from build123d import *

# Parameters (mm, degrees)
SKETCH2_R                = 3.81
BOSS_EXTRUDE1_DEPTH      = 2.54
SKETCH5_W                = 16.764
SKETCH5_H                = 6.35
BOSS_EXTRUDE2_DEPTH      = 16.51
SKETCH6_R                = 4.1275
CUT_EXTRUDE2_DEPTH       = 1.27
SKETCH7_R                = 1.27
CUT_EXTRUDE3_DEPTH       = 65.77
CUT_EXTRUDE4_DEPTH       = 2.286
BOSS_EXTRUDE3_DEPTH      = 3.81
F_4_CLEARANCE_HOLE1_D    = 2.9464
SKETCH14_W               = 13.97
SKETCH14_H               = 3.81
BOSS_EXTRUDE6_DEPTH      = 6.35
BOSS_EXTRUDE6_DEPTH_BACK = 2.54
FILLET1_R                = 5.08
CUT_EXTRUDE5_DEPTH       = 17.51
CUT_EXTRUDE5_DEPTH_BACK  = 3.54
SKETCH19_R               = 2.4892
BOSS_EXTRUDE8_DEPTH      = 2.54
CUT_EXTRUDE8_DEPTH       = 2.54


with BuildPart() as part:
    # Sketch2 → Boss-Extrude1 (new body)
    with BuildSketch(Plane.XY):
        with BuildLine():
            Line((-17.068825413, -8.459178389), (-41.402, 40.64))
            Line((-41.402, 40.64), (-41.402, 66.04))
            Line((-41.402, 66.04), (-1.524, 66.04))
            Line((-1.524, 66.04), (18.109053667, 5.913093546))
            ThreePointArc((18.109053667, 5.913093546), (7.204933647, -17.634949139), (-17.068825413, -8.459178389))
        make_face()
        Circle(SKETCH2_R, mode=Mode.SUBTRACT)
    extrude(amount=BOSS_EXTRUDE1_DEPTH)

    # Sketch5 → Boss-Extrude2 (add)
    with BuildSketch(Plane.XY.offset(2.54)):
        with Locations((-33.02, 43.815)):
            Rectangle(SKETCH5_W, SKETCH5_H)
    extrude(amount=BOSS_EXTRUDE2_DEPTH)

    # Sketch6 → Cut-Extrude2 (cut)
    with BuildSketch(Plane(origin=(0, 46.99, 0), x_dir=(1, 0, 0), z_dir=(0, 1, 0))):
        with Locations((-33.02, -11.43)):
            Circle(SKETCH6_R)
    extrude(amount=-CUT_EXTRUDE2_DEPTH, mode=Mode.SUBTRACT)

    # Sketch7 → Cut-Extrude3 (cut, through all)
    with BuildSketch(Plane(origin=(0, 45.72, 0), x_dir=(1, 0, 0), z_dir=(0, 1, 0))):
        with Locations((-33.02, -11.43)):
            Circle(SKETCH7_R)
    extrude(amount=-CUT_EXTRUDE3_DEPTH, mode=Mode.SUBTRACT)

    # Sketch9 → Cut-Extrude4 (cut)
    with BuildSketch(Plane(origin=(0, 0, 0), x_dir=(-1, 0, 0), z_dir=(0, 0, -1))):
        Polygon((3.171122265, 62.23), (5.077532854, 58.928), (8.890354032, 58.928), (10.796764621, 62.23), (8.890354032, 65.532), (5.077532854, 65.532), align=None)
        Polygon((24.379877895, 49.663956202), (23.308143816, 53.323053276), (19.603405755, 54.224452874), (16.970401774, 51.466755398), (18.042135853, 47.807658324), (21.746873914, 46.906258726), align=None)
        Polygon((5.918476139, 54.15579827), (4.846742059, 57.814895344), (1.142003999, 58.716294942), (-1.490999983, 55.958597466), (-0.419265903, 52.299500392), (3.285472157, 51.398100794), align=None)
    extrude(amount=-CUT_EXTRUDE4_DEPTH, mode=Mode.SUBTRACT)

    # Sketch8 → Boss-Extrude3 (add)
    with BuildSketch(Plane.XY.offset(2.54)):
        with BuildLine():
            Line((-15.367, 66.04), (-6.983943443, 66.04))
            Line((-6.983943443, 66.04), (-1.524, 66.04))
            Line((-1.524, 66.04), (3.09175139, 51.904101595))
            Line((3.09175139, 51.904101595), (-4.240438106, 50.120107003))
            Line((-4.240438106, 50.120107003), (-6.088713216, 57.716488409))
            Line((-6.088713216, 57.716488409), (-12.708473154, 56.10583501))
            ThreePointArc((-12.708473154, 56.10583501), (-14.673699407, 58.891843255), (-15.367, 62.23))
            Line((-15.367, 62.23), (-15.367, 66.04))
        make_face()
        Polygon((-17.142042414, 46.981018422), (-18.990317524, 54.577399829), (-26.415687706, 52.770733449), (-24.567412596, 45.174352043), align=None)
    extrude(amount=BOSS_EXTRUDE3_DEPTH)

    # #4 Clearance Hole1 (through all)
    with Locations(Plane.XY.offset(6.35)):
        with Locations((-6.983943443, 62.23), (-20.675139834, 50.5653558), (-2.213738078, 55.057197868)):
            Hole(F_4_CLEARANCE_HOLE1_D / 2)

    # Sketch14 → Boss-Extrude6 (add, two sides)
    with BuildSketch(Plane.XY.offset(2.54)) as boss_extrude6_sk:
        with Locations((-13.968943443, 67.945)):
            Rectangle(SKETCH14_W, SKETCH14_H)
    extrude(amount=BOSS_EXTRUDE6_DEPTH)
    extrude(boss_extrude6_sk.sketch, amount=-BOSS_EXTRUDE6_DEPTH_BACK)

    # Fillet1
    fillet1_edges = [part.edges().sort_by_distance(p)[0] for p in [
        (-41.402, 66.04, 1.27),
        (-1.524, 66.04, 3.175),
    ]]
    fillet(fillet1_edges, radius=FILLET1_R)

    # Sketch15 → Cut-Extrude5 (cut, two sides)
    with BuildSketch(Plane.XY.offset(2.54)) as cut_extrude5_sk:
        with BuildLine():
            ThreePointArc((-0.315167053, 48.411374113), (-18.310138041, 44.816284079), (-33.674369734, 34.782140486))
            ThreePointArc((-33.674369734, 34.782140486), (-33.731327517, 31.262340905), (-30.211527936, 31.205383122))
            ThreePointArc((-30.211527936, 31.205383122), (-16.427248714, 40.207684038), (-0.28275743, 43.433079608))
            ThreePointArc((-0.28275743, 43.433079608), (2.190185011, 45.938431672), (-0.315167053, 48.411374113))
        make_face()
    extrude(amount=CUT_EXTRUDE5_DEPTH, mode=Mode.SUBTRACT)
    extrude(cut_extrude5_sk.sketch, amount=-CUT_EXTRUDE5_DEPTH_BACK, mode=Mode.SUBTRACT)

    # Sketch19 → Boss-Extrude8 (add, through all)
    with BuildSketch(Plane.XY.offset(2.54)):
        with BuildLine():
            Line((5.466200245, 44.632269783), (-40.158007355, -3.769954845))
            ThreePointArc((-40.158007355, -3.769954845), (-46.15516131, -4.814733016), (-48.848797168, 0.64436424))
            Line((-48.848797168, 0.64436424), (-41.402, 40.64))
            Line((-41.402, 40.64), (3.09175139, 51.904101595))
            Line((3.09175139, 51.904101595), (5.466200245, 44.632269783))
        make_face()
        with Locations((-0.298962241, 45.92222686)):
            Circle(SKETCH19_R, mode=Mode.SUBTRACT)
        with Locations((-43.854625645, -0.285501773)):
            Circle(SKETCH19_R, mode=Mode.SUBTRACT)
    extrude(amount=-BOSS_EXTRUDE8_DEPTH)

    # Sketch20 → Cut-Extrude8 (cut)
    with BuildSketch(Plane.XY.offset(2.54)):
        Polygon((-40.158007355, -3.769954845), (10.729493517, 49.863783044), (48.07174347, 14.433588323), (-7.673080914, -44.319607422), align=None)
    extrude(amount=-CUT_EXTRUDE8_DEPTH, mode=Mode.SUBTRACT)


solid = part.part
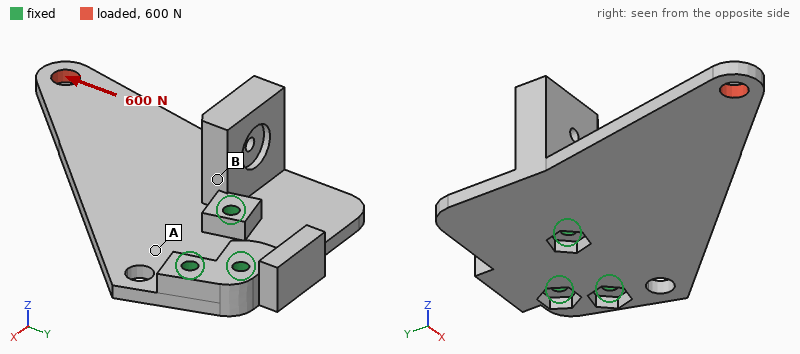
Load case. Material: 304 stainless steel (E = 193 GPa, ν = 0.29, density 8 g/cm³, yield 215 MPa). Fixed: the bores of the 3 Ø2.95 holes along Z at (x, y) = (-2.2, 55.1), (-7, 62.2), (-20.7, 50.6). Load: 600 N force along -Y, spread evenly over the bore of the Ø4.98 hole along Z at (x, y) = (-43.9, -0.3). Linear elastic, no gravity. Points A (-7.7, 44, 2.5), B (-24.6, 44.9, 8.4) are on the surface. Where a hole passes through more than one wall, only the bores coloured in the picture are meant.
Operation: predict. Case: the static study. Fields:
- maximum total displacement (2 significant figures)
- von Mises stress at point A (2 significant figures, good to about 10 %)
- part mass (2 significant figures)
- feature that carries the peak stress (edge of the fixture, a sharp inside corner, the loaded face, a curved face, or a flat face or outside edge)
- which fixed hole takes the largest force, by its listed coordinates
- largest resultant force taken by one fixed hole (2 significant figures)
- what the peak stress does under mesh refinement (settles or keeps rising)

45 µm
22 MPa
67 g
edge of the fixture
(-20.7, 50.6)
970 N
keeps rising
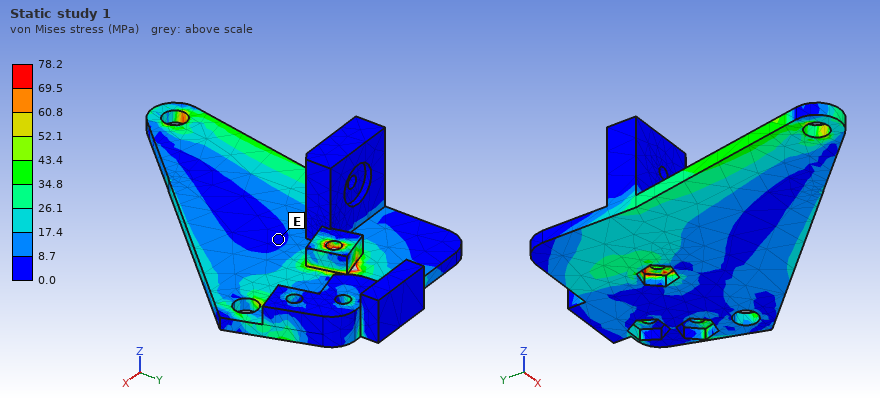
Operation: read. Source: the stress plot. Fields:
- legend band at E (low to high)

0.0 to 8.7 MPa
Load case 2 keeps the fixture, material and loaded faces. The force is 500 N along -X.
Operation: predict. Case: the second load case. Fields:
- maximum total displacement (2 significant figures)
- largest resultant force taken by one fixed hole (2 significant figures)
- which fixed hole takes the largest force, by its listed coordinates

59 µm
1.2 kN
(-20.7, 50.6)
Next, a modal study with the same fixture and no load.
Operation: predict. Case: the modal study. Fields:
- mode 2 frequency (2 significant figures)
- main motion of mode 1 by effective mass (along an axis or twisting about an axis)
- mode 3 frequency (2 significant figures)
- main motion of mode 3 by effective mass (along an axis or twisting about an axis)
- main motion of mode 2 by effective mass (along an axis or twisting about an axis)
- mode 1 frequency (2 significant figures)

3500 Hz
along Z
3900 Hz
along Z
twisting about Y
1100 Hz
